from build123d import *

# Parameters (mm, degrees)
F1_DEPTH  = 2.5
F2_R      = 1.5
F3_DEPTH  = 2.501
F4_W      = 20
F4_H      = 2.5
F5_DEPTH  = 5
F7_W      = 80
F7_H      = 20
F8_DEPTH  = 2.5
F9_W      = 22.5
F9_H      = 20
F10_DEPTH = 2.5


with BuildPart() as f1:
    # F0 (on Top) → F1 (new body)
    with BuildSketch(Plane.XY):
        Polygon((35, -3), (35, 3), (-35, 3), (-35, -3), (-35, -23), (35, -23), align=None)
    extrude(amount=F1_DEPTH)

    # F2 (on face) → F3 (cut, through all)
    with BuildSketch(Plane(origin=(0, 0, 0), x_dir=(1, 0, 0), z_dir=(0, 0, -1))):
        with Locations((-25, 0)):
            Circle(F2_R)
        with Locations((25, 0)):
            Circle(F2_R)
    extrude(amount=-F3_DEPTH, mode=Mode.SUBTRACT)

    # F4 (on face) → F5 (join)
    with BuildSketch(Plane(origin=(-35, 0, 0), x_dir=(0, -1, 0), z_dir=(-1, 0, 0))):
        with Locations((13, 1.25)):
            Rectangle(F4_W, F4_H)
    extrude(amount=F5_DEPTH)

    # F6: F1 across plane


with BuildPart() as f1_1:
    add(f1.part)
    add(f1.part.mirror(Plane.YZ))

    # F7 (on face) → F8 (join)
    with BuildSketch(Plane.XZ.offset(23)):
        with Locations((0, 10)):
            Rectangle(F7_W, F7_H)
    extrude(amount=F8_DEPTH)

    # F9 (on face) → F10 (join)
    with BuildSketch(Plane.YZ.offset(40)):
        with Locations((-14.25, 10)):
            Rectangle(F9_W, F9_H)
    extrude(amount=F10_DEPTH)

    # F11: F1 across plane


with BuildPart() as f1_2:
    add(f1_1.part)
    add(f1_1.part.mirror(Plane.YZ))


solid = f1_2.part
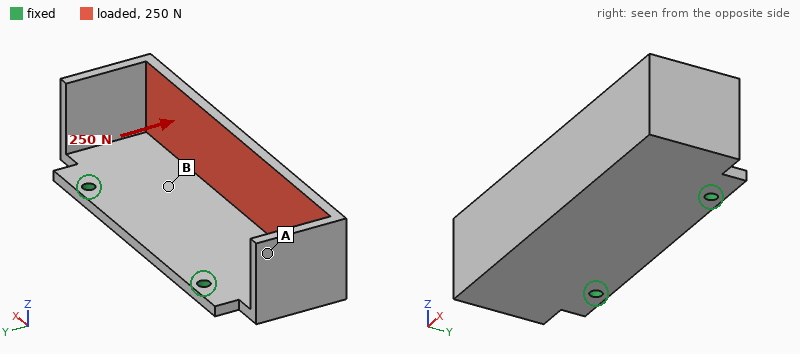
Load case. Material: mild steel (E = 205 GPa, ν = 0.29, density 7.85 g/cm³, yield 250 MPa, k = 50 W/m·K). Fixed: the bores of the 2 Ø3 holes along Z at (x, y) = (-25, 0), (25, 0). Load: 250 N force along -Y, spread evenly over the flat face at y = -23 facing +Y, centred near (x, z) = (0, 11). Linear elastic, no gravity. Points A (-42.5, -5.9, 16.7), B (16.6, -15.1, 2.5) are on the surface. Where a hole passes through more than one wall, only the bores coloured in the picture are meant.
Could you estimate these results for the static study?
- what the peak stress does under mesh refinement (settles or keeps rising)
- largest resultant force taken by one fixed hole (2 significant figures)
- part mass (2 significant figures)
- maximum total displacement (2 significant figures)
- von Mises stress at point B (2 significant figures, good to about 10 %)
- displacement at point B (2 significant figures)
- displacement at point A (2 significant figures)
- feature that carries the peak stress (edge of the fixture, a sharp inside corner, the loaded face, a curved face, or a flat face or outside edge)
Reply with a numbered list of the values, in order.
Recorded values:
1. keeps rising
2. 130 N
3. 88 g
4. 83 µm
5. 21 MPa
6. 23 µm
7. 41 µm
8. edge of the fixture
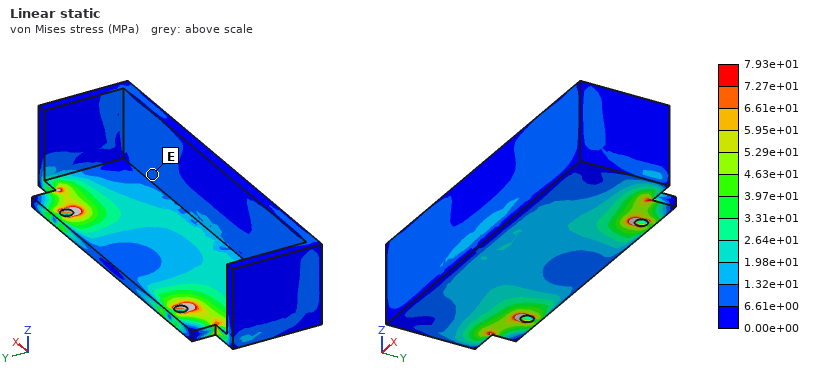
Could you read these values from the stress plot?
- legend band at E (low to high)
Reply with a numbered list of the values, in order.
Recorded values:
1. 6.61e+00 to 1.32e+01 MPa
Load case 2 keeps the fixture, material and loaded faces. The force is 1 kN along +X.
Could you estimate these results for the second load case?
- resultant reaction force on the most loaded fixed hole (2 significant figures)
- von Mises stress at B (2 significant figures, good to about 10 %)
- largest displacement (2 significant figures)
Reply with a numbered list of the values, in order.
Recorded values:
1. 690 N
2. 57 MPa
3. 0.14 mm
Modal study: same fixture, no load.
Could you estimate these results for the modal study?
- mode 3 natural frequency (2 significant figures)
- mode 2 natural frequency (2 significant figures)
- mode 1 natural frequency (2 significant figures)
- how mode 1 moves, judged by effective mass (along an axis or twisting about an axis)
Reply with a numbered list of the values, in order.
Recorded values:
1. 4000 Hz
2. 1500 Hz
3. 1100 Hz
4. along Z
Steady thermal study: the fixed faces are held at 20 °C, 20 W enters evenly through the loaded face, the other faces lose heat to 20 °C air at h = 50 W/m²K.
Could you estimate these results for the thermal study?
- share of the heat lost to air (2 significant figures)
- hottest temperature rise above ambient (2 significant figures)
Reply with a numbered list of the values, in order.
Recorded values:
1. 56 %
2. 50 K
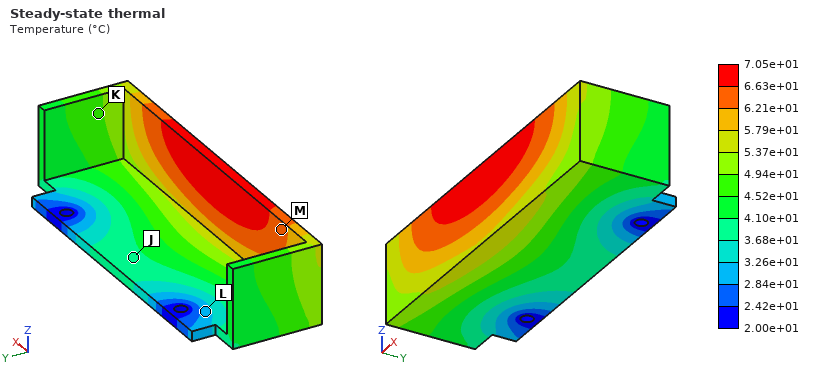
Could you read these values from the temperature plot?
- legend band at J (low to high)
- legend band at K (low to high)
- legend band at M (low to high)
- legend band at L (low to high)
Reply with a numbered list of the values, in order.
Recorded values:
1. 3.68e+01 to 4.10e+01 °C
2. 4.52e+01 to 4.94e+01 °C
3. 6.21e+01 to 6.63e+01 °C
4. 2.84e+01 to 3.26e+01 °C
